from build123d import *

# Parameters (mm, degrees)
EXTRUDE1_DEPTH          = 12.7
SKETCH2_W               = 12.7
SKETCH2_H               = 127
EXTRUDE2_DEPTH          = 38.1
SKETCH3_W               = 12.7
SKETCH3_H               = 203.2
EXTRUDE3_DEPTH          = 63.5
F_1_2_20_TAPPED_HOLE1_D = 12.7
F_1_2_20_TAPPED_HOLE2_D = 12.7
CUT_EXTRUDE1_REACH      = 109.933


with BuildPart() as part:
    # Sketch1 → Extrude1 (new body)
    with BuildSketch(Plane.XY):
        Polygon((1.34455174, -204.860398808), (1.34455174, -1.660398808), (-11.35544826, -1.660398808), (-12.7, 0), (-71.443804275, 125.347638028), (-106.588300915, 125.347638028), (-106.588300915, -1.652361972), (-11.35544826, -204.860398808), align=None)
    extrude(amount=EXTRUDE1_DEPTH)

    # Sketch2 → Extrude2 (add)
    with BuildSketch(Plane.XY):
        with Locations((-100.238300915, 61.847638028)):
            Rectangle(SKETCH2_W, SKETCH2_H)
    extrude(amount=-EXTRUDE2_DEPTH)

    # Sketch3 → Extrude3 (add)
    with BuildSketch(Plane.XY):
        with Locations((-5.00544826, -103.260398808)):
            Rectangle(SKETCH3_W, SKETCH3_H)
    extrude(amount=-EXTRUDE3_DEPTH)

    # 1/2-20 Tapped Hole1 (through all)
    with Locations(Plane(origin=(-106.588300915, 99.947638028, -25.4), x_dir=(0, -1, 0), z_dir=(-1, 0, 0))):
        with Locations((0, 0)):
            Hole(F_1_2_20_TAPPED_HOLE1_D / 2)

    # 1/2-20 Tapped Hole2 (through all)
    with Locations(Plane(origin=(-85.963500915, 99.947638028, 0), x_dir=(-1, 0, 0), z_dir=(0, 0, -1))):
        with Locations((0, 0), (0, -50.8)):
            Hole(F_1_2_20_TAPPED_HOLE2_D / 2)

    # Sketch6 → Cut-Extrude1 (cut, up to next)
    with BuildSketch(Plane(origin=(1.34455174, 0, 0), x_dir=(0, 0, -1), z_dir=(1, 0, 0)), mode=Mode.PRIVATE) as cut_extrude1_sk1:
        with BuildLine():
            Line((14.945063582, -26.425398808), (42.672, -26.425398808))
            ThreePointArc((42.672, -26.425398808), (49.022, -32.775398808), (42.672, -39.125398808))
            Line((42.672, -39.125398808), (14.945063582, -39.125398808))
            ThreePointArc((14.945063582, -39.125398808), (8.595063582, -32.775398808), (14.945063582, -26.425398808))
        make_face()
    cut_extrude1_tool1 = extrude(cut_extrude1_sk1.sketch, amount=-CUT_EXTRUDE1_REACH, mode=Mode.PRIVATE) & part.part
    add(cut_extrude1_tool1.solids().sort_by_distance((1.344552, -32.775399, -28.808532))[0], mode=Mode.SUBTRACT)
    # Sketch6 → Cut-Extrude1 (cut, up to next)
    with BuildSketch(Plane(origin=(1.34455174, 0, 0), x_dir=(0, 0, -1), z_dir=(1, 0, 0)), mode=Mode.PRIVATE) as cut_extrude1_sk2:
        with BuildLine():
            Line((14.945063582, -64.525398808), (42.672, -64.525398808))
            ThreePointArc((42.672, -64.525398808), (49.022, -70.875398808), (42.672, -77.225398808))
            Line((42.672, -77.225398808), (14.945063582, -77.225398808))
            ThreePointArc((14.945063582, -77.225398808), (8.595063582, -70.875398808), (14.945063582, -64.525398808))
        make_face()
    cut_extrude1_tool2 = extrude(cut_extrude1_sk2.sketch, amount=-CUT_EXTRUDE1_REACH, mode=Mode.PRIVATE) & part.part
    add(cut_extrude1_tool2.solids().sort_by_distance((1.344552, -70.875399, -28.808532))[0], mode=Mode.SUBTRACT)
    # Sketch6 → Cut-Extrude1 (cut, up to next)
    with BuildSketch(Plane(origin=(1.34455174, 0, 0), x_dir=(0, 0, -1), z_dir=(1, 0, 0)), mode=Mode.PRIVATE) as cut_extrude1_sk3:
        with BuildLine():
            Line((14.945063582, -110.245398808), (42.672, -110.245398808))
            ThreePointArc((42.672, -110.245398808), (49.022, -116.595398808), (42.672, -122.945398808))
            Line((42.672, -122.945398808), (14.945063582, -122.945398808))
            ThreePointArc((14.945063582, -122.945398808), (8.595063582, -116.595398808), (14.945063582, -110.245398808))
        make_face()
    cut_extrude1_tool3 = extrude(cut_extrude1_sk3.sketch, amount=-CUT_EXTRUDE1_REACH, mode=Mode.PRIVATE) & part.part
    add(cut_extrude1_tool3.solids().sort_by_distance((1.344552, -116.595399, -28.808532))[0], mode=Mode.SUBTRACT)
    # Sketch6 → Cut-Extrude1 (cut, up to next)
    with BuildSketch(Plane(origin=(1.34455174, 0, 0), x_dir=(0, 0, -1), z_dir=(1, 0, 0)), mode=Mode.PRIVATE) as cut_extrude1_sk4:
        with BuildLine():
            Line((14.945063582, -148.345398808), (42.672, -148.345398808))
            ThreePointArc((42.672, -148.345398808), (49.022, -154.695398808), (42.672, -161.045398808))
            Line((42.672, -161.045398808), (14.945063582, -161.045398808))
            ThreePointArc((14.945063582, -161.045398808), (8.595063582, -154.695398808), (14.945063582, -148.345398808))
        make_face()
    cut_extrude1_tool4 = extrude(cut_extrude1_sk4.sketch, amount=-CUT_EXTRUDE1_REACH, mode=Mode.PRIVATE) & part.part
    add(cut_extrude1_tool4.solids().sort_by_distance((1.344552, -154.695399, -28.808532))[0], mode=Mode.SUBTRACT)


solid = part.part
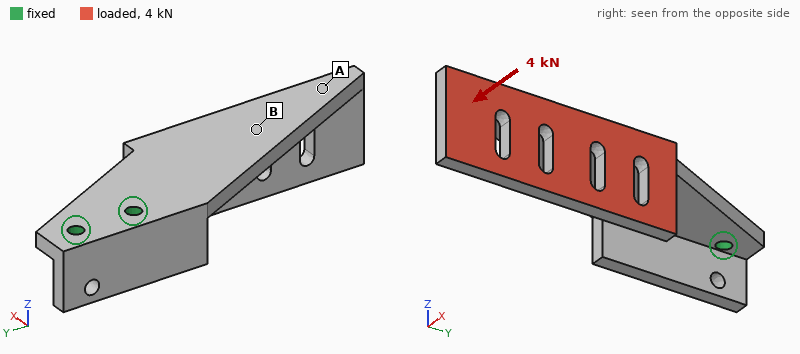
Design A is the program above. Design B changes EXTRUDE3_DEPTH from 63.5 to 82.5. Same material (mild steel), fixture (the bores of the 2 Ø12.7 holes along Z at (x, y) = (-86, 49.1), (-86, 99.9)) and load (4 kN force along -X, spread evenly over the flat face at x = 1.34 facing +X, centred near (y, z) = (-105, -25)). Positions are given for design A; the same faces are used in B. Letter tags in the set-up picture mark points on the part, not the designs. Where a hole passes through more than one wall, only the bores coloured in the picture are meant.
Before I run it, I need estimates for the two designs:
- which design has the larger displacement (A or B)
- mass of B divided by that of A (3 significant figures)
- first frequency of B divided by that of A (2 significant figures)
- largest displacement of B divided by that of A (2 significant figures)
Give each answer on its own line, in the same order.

B
1.11
0.89
1.4
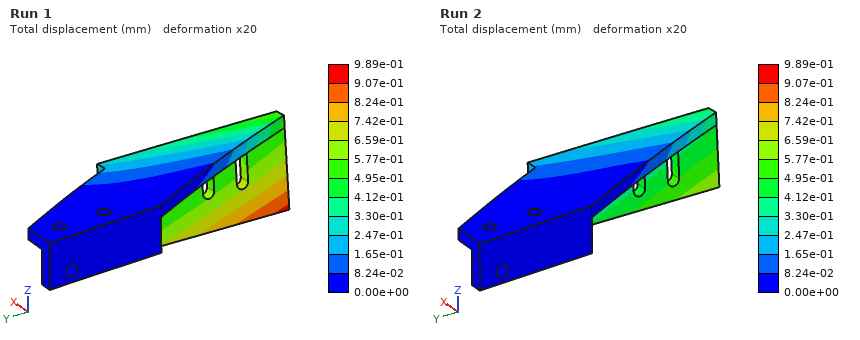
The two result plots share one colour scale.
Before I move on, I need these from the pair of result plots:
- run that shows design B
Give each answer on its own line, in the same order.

Run 1
